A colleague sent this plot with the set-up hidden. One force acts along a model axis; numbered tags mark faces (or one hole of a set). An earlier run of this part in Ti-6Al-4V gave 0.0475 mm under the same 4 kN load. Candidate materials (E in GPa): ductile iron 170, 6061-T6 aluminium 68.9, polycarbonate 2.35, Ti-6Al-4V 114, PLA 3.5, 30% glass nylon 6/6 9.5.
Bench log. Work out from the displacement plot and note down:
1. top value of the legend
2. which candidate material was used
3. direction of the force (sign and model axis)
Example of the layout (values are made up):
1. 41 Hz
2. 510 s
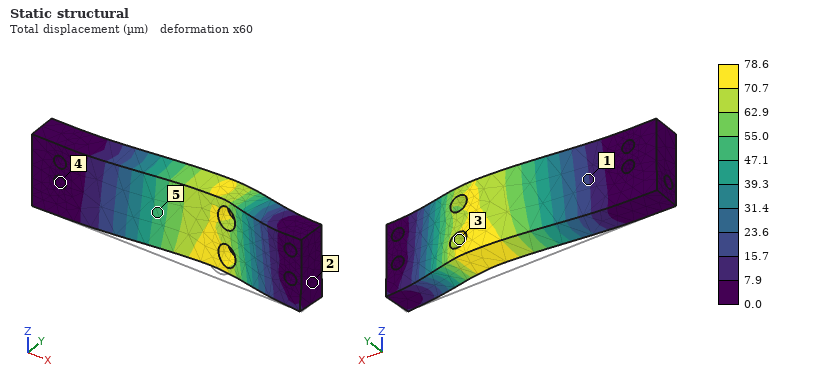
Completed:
1. 78.6 µm
2. 6061-T6 aluminium
3. +Y
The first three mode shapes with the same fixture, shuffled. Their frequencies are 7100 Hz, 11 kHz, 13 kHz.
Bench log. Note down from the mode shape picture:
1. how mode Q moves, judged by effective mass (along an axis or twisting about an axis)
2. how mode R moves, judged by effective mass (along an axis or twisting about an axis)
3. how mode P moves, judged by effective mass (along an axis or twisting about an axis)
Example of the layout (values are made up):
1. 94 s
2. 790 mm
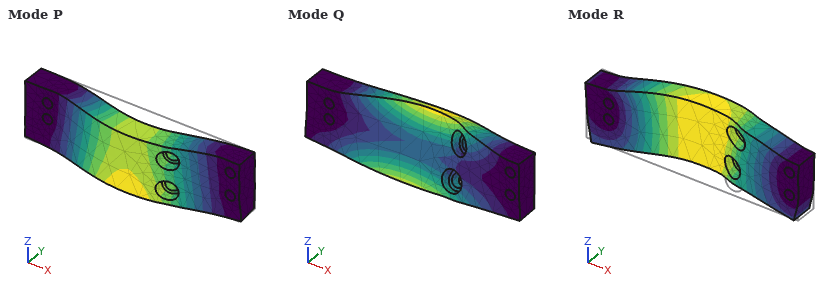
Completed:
1. twisting about X
2. along Z
3. along Y
